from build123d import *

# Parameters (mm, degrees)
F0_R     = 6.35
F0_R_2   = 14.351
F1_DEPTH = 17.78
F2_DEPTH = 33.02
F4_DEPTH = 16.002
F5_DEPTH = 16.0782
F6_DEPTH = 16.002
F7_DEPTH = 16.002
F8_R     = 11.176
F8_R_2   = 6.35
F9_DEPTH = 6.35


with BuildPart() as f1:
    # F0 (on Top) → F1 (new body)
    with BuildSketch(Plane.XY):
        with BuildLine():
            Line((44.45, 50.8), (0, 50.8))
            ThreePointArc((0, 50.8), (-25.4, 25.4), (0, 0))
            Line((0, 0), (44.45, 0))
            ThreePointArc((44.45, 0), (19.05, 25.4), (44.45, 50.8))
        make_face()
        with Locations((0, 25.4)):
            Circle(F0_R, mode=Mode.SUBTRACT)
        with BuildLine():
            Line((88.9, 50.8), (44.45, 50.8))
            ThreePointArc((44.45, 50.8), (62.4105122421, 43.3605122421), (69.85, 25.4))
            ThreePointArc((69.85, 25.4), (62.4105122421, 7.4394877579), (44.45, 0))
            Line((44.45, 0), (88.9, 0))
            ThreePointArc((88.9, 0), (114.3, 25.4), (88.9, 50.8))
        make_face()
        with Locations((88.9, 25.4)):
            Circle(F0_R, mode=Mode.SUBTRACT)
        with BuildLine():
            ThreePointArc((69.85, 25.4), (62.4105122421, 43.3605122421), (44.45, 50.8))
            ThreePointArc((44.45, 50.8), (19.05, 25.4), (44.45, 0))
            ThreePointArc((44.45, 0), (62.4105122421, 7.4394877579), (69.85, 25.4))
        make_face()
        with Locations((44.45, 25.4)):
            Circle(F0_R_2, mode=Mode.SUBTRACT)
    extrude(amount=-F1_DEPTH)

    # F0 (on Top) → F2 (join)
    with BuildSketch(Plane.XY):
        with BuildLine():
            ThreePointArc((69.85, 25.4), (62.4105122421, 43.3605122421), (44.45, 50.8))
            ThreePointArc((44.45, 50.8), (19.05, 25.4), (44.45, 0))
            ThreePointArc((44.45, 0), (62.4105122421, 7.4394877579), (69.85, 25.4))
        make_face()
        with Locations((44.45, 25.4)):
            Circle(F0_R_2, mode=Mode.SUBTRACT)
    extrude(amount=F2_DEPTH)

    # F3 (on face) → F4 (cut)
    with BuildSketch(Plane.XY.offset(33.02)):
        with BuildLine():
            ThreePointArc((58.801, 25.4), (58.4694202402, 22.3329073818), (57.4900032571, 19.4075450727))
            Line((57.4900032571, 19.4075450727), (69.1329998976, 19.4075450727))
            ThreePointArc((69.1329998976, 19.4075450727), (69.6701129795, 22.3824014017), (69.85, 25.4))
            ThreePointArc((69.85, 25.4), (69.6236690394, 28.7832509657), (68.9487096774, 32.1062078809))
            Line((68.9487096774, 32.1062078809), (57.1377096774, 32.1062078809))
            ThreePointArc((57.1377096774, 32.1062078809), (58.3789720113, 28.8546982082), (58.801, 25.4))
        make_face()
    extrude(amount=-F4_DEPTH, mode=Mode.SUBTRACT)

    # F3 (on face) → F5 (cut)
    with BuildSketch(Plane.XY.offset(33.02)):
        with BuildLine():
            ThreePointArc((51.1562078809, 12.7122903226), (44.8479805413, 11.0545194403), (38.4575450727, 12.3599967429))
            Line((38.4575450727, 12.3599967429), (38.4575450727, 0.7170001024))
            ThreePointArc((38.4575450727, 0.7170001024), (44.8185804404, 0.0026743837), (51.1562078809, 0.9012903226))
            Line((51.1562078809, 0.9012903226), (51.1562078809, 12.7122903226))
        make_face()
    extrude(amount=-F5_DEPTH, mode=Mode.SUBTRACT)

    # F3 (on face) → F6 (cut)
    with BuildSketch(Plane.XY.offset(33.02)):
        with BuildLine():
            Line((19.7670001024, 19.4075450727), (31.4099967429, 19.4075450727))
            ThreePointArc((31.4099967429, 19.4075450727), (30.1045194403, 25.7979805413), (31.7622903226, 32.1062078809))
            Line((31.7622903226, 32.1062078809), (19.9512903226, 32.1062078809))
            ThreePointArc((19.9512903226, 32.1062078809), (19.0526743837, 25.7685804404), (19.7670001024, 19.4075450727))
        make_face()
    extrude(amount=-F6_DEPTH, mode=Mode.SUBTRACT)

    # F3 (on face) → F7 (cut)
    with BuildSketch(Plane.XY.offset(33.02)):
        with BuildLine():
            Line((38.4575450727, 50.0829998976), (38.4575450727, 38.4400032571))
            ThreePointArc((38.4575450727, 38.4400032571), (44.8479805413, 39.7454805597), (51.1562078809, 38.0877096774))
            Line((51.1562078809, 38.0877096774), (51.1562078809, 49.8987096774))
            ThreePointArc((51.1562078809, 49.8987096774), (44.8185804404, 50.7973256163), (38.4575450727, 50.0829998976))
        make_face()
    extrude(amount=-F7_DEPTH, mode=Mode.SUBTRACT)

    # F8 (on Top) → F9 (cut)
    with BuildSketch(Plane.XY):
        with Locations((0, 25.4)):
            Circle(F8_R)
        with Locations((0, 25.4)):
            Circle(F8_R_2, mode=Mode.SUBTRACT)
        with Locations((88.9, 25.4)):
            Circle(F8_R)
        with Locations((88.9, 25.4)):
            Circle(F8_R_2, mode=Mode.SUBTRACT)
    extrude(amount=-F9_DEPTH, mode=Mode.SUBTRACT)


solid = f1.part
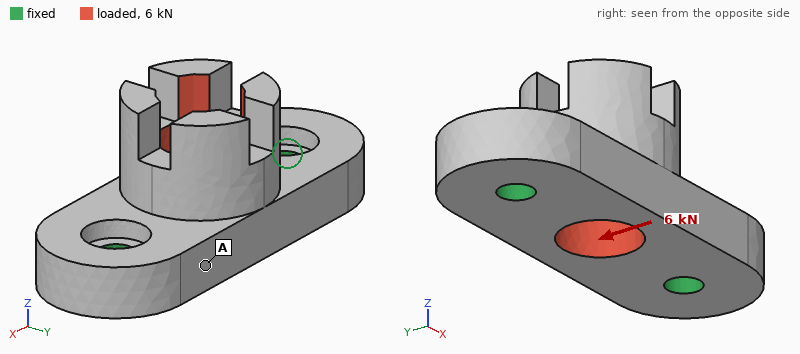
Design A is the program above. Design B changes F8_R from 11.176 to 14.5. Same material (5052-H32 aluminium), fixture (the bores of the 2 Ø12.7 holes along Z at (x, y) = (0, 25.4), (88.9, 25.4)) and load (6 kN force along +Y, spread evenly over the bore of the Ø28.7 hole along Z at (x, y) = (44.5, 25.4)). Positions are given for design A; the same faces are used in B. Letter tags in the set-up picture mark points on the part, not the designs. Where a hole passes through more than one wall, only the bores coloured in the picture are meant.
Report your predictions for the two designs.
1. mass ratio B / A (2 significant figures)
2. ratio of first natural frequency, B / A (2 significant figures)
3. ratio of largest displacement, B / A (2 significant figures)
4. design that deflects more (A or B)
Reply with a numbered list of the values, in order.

1. 0.97
2. 0.96
3. 1.1
4. B
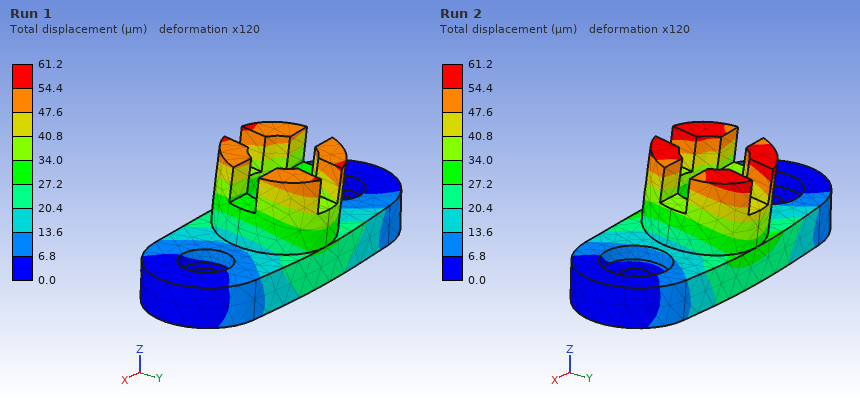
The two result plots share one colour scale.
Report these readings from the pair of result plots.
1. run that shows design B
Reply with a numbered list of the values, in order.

1. Run 2
